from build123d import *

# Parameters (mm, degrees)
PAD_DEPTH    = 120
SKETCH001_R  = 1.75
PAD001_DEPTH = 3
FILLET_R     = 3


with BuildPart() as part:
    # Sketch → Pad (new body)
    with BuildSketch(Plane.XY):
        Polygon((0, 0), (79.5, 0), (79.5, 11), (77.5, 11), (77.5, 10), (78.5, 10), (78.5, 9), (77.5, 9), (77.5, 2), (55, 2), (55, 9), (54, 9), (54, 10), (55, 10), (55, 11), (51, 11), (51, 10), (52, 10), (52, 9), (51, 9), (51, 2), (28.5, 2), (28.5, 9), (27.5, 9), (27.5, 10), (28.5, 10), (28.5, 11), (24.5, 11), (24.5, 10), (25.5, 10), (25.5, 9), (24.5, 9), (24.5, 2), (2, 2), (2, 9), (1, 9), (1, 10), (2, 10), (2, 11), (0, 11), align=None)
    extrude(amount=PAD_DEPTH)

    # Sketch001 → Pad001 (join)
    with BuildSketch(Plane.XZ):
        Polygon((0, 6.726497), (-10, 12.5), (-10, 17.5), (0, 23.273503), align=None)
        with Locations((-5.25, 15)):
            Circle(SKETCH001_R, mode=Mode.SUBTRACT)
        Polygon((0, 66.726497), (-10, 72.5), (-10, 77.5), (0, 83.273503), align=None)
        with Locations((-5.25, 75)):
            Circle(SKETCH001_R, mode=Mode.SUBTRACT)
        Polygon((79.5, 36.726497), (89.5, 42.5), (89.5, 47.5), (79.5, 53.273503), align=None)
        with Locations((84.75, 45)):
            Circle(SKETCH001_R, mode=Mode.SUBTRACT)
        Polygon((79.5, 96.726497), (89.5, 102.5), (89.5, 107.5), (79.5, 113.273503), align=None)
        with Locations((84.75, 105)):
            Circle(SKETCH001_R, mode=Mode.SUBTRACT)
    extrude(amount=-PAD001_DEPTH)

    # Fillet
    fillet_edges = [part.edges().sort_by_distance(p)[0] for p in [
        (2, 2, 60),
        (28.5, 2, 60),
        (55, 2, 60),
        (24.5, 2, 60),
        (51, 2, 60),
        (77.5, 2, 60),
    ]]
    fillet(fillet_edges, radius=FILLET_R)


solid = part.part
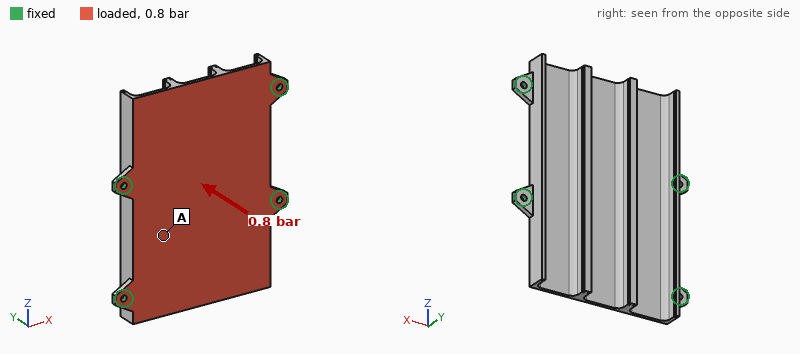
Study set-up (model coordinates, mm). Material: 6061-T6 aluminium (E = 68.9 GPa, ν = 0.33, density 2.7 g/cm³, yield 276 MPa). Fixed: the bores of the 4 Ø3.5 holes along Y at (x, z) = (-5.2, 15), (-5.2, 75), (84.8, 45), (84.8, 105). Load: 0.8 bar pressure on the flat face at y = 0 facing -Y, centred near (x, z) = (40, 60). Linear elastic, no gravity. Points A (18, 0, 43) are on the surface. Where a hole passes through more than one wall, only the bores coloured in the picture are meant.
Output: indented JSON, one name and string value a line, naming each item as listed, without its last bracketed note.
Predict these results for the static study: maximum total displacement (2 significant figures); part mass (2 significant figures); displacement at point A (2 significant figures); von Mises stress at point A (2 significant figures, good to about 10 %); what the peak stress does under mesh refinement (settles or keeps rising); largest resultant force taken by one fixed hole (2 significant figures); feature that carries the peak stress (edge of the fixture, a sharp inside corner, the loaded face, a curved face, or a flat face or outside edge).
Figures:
{
  "maximum total displacement": "0.30 mm",
  "part mass": "91 g",
  "displacement at point A": "0.17 mm",
  "von Mises stress at point A": "15 MPa",
  "what the peak stress does under mesh refinement": "keeps rising",
  "largest resultant force taken by one fixed hole": "400 N",
  "feature that carries the peak stress": "edge of the fixture"
}
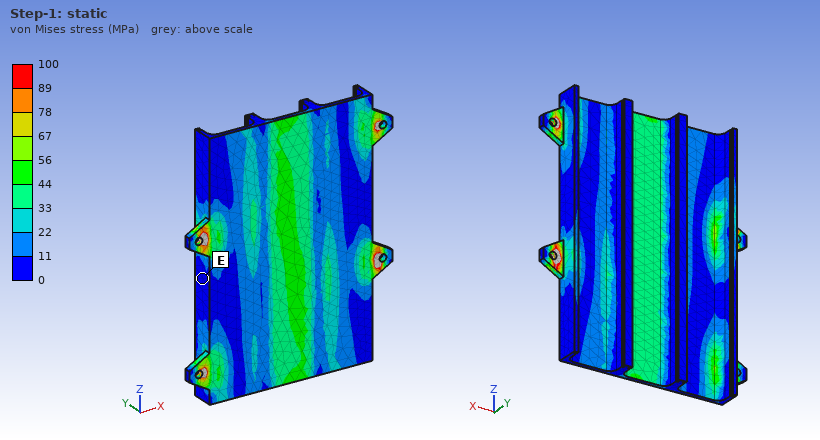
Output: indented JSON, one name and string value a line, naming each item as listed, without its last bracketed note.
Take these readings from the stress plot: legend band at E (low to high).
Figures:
{
  "legend band at E": "0 to 11 MPa"
}
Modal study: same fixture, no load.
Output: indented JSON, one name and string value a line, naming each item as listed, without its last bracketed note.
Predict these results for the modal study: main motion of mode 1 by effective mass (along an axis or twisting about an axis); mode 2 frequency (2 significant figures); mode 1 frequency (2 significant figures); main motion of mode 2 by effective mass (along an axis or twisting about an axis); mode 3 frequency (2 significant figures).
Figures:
{
  "main motion of mode 1 by effective mass": "along Y",
  "mode 2 frequency": "1200 Hz",
  "mode 1 frequency": "990 Hz",
  "main motion of mode 2 by effective mass": "twisting about X",
  "mode 3 frequency": "2600 Hz"
}
